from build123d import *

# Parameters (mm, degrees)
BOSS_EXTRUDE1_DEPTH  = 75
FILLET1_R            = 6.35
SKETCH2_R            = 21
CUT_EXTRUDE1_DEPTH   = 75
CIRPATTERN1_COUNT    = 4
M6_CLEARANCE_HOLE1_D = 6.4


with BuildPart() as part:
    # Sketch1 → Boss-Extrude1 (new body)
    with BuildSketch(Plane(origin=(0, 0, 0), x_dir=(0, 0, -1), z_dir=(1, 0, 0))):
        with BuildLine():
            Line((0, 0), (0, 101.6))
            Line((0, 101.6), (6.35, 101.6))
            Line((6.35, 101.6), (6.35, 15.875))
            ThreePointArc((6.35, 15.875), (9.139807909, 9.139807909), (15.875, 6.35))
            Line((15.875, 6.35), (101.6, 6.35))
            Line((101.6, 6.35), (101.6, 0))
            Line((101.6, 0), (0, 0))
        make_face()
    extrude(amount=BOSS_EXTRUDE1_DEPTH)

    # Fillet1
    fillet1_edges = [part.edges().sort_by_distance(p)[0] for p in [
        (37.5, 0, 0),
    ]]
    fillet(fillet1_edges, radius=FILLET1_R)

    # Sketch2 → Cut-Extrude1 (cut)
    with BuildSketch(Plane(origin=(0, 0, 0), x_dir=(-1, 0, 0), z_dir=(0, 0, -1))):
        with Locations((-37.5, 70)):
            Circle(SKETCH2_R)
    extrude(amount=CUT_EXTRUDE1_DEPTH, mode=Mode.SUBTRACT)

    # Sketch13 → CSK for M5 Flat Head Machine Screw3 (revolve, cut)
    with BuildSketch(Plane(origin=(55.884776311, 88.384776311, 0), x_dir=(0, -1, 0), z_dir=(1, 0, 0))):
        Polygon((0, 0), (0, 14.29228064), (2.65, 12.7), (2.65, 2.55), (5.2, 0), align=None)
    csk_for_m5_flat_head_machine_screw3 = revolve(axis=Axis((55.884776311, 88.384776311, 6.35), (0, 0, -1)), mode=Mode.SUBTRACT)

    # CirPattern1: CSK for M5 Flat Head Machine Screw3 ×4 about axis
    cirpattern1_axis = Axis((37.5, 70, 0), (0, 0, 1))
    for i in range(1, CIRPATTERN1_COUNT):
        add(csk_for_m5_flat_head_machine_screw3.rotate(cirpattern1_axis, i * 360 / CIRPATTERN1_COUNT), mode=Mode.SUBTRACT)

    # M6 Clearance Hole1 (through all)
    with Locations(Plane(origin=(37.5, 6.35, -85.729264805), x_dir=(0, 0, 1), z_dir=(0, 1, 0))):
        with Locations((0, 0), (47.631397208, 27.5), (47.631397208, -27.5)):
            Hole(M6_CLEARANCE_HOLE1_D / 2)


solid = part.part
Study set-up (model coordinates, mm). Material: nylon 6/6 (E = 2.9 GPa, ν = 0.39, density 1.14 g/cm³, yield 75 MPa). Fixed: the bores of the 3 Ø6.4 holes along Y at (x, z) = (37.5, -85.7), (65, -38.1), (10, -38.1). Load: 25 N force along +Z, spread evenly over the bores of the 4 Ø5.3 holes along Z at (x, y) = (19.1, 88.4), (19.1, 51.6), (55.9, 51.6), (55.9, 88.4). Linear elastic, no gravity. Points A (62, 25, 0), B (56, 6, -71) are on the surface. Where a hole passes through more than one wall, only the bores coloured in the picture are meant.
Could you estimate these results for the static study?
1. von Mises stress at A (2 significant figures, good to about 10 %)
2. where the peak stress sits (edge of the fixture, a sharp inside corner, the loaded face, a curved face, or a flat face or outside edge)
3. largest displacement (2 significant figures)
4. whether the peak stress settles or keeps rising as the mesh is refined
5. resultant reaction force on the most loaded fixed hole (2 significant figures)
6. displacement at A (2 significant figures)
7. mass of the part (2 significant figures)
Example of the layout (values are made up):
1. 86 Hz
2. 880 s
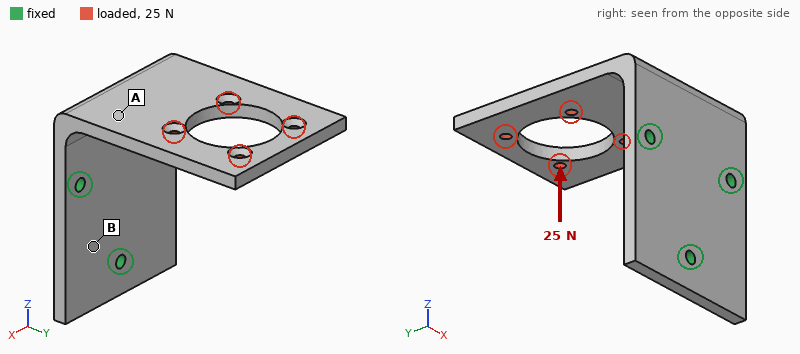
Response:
1. 2.0 MPa
2. edge of the fixture
3. 1.8 mm
4. keeps rising
5. 13 N
6. 0.35 mm
7. 96 g
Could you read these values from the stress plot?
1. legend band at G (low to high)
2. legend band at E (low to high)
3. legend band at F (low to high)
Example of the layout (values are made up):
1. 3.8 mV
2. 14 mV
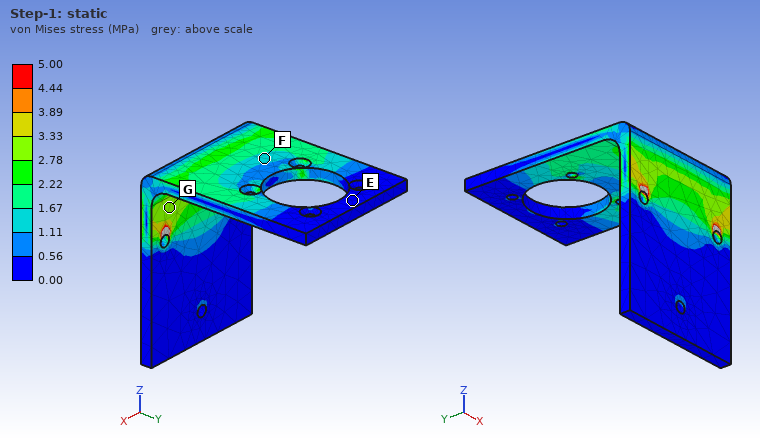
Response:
1. 2.78 to 3.33 MPa
2. 0.00 to 0.56 MPa
3. 1.11 to 1.67 MPa
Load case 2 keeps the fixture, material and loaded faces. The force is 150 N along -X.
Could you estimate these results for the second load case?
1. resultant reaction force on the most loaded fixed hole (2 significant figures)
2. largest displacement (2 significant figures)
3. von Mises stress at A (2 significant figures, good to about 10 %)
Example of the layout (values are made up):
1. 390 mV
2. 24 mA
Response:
1. 210 N
2. 1.7 mm
3. 2.4 MPa
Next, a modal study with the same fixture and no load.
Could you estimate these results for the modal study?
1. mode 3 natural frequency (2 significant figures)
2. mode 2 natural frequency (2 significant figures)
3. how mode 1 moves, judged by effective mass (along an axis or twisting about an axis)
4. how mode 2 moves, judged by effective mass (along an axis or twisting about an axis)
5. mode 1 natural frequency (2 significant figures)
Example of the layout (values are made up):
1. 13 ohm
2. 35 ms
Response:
1. 460 Hz
2. 320 Hz
3. along Z
4. along X
5. 140 Hz
